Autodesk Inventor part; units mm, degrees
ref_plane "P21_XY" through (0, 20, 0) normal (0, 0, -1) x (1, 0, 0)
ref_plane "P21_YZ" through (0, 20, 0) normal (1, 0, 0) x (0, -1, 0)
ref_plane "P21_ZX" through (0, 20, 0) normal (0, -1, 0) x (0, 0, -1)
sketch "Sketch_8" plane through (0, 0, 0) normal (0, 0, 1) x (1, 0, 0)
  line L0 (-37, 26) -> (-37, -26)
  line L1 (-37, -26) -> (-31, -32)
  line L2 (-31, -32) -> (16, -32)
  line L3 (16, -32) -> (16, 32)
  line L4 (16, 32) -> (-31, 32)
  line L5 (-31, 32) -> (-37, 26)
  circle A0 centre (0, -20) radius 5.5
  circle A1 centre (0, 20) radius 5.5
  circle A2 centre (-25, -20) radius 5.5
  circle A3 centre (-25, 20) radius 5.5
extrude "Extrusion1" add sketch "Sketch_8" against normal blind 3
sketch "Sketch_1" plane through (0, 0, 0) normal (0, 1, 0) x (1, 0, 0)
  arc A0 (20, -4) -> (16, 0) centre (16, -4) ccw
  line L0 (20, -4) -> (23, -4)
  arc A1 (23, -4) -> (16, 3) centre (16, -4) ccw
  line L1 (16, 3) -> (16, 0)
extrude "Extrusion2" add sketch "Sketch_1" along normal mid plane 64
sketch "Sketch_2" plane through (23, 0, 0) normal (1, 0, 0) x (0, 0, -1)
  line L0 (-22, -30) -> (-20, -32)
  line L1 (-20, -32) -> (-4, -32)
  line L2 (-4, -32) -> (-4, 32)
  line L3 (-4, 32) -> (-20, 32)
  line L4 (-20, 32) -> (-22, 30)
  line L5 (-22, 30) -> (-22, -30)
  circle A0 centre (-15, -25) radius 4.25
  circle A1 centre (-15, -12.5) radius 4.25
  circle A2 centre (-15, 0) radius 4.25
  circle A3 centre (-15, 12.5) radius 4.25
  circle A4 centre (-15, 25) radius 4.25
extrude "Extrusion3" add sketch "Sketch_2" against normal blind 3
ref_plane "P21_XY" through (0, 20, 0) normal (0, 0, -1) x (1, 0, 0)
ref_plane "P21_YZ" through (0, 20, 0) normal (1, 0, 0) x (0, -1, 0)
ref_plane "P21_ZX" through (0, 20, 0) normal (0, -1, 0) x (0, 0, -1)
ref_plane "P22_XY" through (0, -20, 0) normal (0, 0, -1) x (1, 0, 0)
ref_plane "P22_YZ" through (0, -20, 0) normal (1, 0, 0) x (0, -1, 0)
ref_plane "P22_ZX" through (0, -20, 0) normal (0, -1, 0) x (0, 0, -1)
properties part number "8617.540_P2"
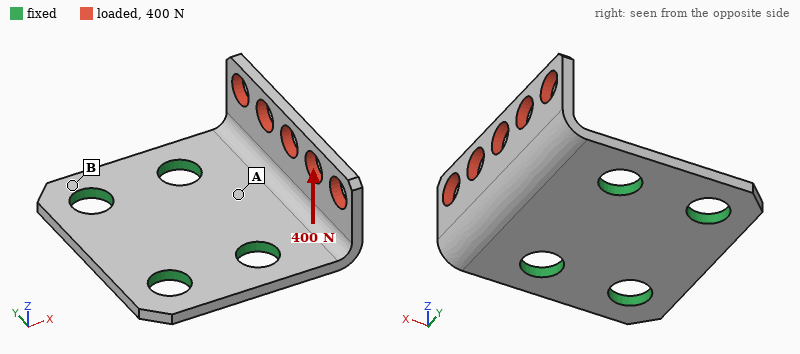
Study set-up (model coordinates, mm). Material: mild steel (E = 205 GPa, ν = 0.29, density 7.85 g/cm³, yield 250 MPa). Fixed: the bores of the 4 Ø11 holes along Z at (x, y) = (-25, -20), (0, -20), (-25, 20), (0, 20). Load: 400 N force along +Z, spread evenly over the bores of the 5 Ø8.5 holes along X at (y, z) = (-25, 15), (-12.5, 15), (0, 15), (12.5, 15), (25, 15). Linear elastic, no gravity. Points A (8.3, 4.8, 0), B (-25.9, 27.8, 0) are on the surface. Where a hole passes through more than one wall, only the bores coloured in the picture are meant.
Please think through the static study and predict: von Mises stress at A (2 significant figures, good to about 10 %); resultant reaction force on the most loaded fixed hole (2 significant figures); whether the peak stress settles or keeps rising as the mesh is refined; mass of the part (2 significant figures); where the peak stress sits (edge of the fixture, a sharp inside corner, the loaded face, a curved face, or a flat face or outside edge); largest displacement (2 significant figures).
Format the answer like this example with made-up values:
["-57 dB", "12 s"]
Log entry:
["33 MPa", "210 N", "keeps rising", "100 g", "edge of the fixture", "59 µm"]
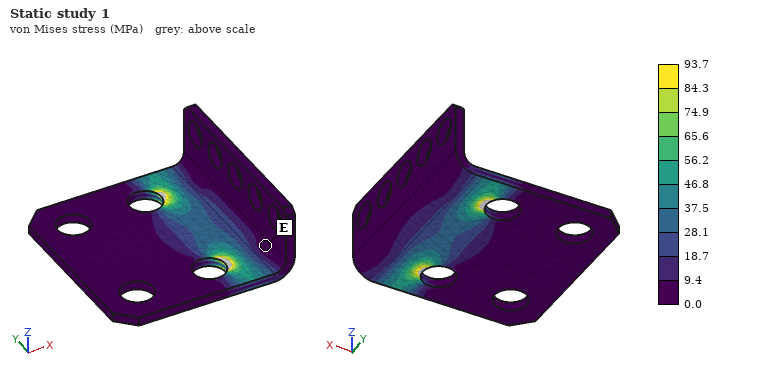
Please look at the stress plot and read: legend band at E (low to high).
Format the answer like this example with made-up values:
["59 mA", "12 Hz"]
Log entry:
["0.0 to 9.4 MPa"]
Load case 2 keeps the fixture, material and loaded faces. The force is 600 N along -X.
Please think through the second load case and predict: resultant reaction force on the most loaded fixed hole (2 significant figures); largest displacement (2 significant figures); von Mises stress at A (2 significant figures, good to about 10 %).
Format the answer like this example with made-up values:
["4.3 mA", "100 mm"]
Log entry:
["260 N", "0.18 mm", "74 MPa"]
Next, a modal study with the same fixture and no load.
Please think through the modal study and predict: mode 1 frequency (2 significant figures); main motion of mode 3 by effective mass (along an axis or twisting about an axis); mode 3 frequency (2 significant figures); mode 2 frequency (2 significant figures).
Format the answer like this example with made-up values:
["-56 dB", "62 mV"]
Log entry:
["2300 Hz", "along Z", "6300 Hz", "3500 Hz"]
